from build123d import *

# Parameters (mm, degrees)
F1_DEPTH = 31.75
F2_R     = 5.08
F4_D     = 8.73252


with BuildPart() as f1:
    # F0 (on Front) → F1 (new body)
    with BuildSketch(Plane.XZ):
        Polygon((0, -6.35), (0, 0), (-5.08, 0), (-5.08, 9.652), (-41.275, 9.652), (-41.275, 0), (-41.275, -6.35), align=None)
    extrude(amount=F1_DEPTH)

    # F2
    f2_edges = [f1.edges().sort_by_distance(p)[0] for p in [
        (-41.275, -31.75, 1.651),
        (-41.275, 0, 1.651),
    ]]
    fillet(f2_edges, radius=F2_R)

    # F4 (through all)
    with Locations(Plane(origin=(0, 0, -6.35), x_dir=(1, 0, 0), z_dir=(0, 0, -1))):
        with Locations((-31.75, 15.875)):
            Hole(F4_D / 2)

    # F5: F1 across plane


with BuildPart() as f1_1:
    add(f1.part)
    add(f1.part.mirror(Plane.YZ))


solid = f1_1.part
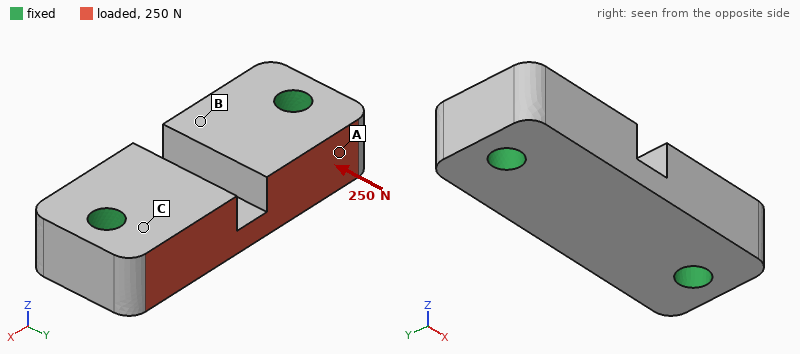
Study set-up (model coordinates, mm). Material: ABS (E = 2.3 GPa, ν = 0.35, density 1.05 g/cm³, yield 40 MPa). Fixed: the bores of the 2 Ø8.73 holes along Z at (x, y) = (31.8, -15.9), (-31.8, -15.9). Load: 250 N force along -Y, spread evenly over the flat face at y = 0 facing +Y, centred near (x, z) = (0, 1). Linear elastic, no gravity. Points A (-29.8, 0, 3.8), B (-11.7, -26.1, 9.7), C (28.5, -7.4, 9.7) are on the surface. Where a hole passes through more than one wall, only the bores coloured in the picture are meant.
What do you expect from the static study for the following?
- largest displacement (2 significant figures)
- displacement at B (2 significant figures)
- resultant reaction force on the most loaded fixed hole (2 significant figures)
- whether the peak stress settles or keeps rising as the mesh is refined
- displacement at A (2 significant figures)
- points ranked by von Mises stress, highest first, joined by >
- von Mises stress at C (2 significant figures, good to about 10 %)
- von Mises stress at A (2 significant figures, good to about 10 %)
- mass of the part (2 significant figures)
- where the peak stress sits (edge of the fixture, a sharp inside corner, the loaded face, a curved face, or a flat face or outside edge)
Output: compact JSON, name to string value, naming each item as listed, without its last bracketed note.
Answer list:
{"largest displacement": "12 µm", "displacement at B": "7.0 µm", "resultant reaction force on the most loaded fixed hole": "130 N", "whether the peak stress settles or keeps rising as the mesh is refined": "keeps rising", "displacement at A": "4.3 µm", "points ranked by von Mises stress, highest first, joined by >": "C > A > B", "von Mises stress at C": "0.43 MPa", "von Mises stress at A": "0.32 MPa", "mass of the part": "38 g", "where the peak stress sits": "edge of the fixture"}
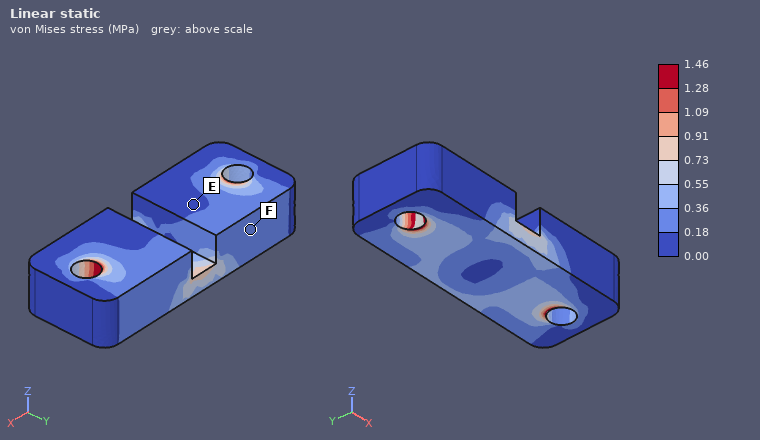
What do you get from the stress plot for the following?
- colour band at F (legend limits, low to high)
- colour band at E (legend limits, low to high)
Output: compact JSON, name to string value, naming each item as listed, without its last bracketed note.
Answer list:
{"colour band at F": "0.18 to 0.36 MPa", "colour band at E": "0.00 to 0.18 MPa"}
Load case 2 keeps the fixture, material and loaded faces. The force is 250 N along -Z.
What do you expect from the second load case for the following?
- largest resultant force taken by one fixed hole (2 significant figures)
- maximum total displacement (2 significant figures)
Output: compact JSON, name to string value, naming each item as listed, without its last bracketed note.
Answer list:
{"largest resultant force taken by one fixed hole": "130 N", "maximum total displacement": "37 µm"}
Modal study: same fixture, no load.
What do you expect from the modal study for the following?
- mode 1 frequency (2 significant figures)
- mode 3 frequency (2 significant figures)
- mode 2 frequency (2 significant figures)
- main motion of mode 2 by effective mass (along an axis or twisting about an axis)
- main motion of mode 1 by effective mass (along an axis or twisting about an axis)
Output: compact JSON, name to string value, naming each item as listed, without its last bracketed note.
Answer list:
{"mode 1 frequency": "4300 Hz", "mode 3 frequency": "5900 Hz", "mode 2 frequency": "4600 Hz", "main motion of mode 2 by effective mass": "along Y", "main motion of mode 1 by effective mass": "along Z"}
